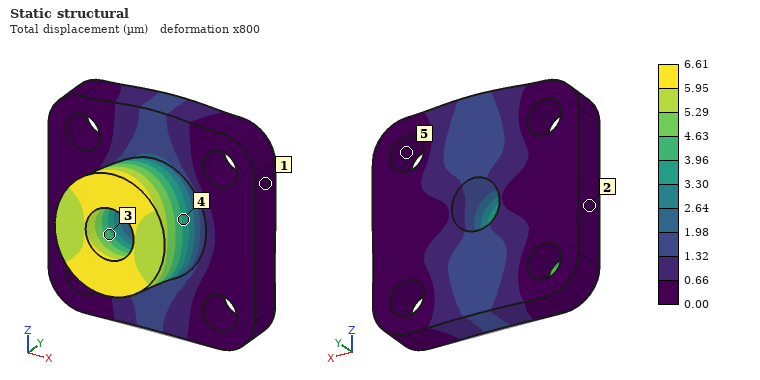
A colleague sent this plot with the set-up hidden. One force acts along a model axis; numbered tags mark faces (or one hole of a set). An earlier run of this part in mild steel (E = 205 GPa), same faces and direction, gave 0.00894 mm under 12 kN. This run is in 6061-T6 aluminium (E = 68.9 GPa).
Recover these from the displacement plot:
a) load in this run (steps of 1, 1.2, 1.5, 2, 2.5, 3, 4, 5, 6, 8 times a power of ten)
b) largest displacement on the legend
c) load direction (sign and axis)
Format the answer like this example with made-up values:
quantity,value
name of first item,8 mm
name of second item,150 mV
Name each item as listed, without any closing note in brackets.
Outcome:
quantity,value
load in this run,3 kN
largest displacement on the legend,6.61 µm
load direction,+Z
